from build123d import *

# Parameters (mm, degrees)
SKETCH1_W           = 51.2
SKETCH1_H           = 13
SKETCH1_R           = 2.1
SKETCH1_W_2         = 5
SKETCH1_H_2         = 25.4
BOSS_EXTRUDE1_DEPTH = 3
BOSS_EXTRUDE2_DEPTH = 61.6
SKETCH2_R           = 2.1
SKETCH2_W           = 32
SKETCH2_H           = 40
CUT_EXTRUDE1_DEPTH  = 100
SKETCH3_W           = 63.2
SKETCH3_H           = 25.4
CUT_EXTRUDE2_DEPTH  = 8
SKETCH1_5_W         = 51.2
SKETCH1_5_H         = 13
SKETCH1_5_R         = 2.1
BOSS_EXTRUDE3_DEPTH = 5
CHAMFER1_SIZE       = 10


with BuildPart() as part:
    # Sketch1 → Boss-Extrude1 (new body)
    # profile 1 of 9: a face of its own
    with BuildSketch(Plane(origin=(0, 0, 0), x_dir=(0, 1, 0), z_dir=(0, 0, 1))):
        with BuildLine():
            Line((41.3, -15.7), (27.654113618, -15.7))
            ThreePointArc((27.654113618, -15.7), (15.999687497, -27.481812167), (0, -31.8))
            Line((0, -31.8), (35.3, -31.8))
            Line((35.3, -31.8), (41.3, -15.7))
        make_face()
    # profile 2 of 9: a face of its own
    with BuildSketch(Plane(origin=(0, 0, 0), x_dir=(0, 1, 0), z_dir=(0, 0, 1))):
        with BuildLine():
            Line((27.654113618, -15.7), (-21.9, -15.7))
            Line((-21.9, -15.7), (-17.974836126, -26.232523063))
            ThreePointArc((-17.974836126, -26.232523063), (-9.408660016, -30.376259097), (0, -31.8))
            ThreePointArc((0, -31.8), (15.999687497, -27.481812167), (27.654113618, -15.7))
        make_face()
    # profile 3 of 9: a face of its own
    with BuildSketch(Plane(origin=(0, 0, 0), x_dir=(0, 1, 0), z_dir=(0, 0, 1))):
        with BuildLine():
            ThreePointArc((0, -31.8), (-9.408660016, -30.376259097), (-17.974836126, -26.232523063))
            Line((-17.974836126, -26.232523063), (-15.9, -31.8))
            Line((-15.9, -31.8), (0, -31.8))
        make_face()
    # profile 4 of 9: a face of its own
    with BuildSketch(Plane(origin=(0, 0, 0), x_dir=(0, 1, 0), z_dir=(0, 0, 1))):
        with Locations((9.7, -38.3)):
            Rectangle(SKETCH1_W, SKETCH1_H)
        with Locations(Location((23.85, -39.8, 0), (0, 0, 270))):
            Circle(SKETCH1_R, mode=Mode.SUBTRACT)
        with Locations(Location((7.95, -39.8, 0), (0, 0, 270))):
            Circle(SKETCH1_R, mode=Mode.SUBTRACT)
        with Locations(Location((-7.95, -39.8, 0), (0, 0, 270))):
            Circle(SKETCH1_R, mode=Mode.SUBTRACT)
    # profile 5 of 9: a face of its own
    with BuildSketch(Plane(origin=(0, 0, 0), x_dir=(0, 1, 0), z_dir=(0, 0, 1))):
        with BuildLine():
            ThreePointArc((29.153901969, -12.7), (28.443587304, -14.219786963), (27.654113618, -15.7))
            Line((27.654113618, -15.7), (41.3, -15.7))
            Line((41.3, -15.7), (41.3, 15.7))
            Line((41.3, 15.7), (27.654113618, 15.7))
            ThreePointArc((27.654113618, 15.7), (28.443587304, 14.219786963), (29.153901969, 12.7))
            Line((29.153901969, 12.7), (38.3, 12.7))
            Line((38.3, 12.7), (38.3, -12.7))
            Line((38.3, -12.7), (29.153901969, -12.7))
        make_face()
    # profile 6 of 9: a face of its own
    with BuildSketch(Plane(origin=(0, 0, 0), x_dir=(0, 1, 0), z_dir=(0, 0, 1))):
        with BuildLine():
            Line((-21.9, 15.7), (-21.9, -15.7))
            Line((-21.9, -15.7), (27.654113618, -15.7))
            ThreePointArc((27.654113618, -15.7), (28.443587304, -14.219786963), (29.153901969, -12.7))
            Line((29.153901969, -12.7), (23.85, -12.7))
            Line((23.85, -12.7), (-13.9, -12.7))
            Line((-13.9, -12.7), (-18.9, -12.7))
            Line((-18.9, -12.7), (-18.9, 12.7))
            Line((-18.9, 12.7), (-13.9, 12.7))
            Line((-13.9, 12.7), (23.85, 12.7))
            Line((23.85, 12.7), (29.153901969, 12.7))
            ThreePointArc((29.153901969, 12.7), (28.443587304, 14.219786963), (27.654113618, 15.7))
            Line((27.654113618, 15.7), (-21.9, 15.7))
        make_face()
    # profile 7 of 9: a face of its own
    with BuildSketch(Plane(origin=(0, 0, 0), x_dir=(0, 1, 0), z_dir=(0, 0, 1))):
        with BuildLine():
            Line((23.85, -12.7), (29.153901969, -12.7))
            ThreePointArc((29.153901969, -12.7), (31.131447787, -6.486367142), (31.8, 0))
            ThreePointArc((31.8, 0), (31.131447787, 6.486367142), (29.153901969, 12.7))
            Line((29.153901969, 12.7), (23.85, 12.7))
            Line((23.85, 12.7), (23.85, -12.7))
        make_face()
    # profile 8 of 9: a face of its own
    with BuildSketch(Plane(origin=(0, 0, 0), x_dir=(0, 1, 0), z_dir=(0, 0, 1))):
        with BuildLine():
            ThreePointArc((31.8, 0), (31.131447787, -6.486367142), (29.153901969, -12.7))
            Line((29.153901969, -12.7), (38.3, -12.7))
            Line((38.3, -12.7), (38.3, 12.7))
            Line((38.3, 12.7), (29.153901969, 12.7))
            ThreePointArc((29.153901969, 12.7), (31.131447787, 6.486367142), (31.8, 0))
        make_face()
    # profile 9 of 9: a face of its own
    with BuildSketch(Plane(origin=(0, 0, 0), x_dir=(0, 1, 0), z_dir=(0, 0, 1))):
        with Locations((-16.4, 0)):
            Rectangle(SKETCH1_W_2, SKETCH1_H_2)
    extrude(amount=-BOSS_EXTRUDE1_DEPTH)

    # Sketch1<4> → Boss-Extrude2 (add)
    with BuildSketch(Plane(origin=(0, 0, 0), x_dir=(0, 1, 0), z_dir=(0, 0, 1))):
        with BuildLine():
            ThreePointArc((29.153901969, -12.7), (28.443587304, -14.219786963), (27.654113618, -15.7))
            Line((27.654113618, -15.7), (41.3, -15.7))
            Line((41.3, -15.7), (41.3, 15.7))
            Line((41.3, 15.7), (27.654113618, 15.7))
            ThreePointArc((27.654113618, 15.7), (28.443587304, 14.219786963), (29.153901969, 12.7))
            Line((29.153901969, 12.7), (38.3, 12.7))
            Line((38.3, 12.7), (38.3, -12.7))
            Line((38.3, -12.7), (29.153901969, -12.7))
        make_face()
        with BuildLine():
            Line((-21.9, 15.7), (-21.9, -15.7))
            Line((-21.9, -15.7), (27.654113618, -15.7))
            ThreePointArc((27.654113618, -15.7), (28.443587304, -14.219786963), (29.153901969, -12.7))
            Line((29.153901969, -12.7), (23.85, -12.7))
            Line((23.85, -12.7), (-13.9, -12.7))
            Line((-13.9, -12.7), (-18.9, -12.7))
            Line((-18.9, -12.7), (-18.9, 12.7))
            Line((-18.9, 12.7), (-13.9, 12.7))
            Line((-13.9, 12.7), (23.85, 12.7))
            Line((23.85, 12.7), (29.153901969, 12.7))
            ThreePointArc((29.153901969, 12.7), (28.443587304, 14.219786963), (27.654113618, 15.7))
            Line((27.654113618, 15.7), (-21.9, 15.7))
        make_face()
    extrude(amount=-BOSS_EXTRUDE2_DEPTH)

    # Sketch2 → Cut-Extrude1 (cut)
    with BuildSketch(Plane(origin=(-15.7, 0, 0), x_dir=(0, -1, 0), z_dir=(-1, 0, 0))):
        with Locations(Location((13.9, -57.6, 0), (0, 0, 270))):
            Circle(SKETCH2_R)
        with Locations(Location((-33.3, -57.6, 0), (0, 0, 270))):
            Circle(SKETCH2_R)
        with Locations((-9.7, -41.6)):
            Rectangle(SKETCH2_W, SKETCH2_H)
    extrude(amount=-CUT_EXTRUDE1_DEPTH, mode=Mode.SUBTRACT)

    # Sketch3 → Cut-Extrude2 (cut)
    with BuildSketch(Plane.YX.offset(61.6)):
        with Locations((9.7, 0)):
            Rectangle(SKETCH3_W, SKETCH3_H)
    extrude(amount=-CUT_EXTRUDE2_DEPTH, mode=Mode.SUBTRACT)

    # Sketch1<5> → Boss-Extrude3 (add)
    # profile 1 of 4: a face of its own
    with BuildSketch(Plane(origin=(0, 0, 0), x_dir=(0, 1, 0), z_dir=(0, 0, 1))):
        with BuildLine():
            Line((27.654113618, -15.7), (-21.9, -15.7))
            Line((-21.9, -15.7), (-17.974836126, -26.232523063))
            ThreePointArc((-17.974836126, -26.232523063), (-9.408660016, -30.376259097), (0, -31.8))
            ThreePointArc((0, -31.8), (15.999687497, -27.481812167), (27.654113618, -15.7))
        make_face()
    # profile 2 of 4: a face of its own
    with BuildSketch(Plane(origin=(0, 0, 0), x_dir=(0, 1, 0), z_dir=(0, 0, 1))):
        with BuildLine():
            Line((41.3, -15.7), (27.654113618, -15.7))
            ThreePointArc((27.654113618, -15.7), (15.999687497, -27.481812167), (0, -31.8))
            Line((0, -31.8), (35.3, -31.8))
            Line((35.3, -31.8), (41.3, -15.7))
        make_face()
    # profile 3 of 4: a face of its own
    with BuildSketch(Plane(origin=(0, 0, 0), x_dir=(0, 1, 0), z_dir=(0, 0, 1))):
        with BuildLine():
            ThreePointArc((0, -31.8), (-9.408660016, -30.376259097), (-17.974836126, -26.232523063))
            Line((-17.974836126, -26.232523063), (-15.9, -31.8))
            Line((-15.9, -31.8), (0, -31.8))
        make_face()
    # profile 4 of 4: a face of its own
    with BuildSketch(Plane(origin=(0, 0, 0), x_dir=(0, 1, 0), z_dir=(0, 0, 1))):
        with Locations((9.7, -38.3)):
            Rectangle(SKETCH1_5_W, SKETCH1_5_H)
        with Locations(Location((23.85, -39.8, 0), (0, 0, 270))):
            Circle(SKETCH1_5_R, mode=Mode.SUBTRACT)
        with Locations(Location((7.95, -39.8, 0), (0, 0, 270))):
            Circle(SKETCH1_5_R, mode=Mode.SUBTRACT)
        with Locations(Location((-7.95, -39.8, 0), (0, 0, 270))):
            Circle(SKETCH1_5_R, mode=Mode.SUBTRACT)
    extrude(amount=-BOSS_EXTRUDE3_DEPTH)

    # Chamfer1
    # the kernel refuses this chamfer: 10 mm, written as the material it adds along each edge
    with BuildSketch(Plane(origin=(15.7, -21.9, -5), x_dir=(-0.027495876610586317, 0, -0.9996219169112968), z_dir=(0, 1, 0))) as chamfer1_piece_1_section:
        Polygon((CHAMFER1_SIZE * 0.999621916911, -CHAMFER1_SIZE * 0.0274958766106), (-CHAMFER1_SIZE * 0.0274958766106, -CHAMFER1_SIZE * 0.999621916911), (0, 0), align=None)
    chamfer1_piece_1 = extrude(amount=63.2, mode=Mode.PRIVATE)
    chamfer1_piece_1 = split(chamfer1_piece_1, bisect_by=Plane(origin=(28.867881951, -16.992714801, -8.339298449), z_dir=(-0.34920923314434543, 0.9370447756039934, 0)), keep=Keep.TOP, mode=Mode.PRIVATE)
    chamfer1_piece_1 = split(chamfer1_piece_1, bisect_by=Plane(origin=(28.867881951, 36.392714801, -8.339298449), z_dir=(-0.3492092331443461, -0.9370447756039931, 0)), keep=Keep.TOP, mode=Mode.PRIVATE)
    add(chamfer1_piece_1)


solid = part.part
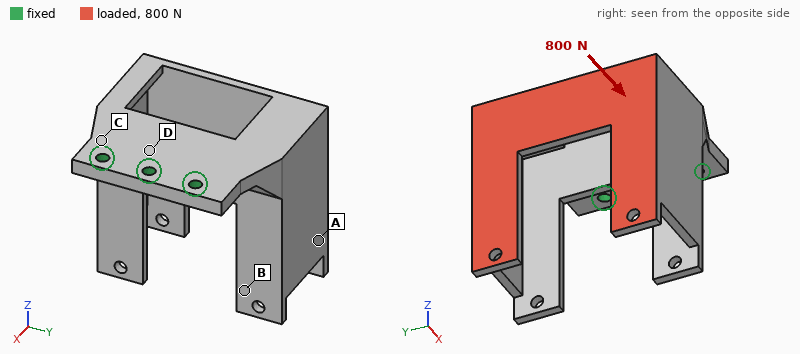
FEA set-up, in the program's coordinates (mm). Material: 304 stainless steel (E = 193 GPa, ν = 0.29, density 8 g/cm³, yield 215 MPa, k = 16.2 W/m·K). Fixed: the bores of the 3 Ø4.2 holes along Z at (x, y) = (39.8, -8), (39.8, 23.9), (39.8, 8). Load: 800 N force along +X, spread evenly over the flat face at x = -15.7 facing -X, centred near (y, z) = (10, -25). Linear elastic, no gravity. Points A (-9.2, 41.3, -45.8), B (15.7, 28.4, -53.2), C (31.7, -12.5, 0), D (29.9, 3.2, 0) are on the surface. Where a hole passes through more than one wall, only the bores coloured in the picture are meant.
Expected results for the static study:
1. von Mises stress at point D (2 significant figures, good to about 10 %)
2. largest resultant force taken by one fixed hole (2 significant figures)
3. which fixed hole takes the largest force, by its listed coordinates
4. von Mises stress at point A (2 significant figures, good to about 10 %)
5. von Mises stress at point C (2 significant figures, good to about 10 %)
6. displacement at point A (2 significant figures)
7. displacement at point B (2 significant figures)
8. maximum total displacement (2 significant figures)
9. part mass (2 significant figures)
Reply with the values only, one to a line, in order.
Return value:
70 MPa
400 N
(39.8, 23.9)
18 MPa
80 MPa
0.20 mm
0.17 mm
0.27 mm
290 g
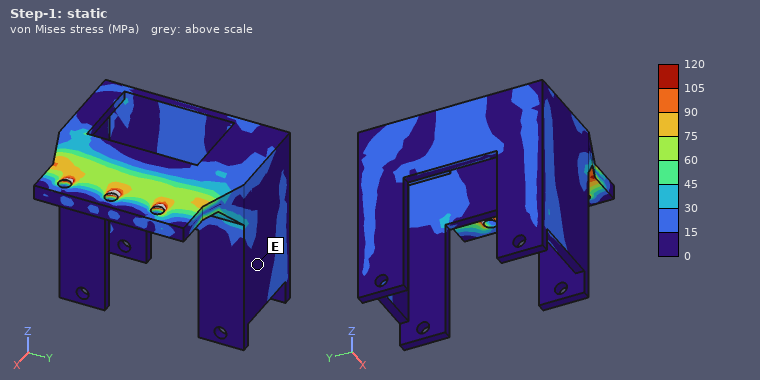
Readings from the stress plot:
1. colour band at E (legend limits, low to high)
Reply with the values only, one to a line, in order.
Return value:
0 to 15 MPa
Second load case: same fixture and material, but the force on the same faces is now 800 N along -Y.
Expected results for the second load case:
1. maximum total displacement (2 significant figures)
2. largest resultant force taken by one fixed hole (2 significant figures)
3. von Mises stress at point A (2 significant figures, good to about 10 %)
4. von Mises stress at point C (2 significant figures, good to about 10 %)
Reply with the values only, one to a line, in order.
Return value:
0.16 mm
1.4 kN
16 MPa
36 MPa
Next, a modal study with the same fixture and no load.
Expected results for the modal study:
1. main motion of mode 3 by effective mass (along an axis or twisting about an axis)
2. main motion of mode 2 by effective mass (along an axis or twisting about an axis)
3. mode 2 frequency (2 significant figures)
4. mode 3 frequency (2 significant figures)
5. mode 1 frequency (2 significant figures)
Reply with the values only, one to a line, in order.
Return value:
along Y
along Y
1100 Hz
2500 Hz
610 Hz
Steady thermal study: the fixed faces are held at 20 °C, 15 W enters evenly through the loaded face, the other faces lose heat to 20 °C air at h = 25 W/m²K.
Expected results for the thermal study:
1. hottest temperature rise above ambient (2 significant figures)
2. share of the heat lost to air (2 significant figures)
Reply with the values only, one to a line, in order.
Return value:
74 K
86 %
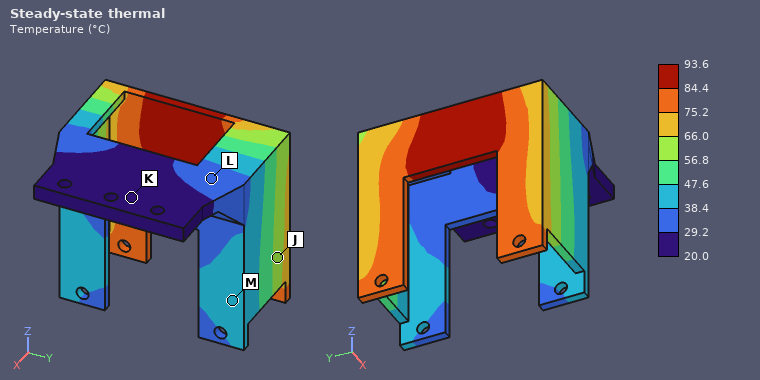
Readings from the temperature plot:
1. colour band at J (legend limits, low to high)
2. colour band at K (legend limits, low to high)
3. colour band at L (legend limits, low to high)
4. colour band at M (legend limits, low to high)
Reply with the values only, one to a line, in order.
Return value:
56.8 to 66.0 °C
20.0 to 29.2 °C
29.2 to 38.4 °C
38.4 to 47.6 °C
